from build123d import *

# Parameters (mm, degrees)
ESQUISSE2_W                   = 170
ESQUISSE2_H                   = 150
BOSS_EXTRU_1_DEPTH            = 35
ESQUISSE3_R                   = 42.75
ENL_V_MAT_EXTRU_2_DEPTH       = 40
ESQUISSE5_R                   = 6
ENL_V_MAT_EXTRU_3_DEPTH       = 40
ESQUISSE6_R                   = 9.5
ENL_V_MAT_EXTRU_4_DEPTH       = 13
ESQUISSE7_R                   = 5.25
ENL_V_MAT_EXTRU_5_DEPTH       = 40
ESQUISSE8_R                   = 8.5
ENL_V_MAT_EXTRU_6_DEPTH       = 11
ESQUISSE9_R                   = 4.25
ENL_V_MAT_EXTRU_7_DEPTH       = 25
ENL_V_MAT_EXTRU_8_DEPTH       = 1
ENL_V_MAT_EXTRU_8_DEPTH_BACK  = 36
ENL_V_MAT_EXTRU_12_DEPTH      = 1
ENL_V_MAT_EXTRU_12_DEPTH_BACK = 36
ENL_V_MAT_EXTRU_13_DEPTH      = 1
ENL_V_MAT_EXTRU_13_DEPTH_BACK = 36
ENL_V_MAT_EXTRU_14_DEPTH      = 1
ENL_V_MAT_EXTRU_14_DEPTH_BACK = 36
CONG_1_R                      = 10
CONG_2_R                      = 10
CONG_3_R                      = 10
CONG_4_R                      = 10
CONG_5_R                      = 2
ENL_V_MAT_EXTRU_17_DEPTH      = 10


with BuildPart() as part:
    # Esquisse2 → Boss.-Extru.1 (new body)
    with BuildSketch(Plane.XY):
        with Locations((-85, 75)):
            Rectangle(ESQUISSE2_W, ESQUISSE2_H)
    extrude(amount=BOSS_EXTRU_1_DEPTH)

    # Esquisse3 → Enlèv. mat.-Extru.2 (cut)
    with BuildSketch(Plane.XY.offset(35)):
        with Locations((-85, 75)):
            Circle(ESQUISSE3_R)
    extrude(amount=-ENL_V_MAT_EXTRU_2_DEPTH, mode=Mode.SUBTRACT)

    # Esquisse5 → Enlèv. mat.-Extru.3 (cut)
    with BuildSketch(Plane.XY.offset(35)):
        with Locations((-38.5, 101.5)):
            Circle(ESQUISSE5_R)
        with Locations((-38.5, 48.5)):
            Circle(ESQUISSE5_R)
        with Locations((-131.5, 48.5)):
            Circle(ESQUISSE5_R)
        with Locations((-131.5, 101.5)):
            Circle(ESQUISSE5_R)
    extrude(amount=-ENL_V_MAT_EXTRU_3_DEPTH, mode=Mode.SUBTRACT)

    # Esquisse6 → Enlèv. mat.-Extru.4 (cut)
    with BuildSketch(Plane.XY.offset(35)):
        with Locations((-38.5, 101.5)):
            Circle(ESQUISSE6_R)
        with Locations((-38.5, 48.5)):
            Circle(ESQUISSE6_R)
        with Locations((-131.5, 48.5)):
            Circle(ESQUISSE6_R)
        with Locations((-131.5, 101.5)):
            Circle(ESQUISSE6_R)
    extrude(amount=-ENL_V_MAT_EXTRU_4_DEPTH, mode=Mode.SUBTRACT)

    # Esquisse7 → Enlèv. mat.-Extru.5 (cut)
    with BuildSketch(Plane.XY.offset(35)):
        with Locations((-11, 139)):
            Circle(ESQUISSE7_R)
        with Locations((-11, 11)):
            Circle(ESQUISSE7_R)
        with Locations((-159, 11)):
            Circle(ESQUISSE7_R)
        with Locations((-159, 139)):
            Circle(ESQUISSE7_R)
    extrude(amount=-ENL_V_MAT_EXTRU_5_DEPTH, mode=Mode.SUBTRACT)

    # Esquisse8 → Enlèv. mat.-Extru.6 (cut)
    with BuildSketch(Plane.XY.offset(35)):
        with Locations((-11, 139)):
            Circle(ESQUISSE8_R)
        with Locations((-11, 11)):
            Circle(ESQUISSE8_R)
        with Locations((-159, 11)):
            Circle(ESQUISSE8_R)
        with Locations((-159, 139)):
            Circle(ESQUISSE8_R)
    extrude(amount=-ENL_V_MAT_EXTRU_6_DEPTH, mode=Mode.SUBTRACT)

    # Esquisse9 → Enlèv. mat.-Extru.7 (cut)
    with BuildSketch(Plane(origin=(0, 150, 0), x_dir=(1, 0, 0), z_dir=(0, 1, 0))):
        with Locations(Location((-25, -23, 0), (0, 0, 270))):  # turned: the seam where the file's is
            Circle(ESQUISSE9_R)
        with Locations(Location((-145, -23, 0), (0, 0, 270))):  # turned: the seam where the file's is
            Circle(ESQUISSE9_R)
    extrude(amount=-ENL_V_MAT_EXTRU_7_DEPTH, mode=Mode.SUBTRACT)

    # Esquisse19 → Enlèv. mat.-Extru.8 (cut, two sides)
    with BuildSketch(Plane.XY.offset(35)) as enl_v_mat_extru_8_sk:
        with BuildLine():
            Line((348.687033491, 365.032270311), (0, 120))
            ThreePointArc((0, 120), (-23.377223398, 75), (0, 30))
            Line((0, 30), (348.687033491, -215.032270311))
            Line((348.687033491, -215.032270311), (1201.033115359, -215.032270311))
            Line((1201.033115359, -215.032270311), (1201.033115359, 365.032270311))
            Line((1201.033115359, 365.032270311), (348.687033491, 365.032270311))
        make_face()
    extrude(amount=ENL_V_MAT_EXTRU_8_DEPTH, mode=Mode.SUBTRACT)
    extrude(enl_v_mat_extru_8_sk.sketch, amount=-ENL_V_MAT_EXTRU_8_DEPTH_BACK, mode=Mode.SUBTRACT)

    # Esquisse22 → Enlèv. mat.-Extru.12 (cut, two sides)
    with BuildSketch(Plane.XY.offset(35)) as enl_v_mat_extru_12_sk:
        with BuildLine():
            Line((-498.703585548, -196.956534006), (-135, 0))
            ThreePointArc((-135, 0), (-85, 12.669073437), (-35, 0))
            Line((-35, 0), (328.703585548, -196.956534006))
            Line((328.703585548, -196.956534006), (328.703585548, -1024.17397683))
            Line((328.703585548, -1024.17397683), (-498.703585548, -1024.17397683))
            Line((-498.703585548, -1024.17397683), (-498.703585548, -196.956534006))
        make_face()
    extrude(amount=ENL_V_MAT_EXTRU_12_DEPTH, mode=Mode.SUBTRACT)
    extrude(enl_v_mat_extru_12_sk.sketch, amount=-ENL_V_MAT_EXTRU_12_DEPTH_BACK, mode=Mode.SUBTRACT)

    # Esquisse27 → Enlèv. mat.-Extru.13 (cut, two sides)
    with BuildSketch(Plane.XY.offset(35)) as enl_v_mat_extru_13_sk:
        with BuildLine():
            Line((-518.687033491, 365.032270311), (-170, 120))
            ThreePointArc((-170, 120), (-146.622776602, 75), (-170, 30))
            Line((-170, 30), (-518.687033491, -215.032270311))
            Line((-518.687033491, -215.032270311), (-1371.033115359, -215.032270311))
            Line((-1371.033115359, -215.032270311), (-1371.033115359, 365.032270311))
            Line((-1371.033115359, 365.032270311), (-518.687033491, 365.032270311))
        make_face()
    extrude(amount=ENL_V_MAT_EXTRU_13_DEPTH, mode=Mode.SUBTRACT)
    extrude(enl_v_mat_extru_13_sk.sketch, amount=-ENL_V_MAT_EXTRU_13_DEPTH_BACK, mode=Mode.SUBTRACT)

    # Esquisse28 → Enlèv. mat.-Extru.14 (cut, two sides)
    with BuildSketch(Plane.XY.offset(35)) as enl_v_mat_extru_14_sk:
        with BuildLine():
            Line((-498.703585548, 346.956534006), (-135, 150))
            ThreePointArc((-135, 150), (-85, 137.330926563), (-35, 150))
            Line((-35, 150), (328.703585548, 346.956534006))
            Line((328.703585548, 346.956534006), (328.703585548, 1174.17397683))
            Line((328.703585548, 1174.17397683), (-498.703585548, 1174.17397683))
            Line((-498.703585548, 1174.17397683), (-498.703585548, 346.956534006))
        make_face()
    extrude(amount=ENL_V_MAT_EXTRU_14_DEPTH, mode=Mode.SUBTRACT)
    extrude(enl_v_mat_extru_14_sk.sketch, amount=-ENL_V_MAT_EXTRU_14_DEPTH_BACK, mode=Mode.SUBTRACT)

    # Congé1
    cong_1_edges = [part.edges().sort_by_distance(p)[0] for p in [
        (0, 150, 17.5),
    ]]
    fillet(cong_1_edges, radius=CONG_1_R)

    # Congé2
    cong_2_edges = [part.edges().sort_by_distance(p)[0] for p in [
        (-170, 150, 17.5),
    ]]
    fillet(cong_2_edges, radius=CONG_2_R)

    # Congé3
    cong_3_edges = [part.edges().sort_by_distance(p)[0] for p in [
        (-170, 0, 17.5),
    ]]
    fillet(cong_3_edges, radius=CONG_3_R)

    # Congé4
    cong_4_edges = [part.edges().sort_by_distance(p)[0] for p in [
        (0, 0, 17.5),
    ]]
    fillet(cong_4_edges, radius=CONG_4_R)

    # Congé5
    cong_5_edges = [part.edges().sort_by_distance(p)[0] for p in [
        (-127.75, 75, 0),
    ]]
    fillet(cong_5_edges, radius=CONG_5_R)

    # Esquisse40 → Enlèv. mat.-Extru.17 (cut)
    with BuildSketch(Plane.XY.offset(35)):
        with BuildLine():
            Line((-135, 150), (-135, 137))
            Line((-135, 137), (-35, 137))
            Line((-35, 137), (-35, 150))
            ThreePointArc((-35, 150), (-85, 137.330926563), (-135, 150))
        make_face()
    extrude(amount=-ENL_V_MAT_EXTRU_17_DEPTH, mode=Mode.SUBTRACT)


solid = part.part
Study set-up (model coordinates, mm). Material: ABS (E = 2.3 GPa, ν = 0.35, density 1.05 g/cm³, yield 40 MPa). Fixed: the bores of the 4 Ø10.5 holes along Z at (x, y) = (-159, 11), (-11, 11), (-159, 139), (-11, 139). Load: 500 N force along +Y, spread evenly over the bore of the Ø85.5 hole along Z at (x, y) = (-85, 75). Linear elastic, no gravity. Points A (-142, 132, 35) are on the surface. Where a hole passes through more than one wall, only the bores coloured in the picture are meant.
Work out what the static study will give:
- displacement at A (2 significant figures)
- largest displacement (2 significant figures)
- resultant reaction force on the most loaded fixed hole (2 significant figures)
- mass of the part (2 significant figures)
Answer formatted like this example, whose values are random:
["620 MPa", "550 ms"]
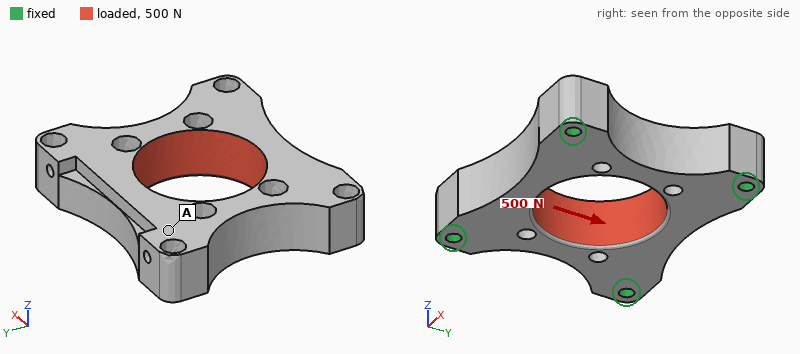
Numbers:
["4.1 µm", "14 µm", "150 N", "500 g"]
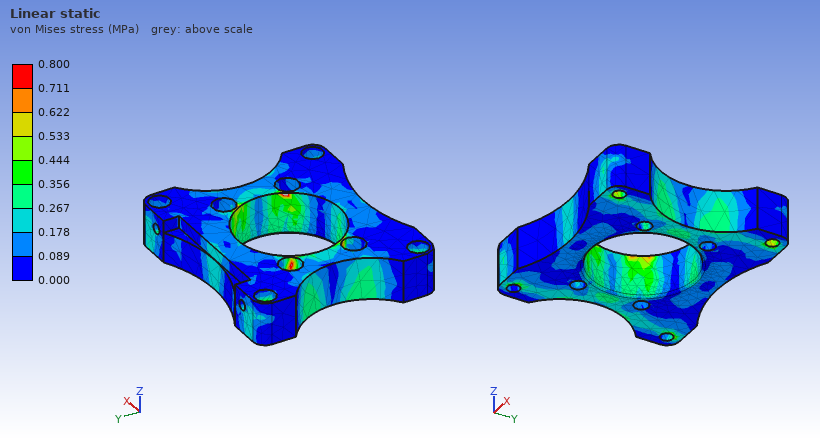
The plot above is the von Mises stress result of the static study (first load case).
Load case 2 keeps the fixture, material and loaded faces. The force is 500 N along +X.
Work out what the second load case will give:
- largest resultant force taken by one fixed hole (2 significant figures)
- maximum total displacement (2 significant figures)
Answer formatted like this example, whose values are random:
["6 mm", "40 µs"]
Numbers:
["150 N", "9.9 µm"]
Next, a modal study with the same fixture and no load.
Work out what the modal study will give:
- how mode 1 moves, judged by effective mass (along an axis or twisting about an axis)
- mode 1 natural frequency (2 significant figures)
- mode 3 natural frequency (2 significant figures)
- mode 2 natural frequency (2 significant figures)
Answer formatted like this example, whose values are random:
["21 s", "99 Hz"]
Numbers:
["along Z", "1300 Hz", "1800 Hz", "1700 Hz"]
